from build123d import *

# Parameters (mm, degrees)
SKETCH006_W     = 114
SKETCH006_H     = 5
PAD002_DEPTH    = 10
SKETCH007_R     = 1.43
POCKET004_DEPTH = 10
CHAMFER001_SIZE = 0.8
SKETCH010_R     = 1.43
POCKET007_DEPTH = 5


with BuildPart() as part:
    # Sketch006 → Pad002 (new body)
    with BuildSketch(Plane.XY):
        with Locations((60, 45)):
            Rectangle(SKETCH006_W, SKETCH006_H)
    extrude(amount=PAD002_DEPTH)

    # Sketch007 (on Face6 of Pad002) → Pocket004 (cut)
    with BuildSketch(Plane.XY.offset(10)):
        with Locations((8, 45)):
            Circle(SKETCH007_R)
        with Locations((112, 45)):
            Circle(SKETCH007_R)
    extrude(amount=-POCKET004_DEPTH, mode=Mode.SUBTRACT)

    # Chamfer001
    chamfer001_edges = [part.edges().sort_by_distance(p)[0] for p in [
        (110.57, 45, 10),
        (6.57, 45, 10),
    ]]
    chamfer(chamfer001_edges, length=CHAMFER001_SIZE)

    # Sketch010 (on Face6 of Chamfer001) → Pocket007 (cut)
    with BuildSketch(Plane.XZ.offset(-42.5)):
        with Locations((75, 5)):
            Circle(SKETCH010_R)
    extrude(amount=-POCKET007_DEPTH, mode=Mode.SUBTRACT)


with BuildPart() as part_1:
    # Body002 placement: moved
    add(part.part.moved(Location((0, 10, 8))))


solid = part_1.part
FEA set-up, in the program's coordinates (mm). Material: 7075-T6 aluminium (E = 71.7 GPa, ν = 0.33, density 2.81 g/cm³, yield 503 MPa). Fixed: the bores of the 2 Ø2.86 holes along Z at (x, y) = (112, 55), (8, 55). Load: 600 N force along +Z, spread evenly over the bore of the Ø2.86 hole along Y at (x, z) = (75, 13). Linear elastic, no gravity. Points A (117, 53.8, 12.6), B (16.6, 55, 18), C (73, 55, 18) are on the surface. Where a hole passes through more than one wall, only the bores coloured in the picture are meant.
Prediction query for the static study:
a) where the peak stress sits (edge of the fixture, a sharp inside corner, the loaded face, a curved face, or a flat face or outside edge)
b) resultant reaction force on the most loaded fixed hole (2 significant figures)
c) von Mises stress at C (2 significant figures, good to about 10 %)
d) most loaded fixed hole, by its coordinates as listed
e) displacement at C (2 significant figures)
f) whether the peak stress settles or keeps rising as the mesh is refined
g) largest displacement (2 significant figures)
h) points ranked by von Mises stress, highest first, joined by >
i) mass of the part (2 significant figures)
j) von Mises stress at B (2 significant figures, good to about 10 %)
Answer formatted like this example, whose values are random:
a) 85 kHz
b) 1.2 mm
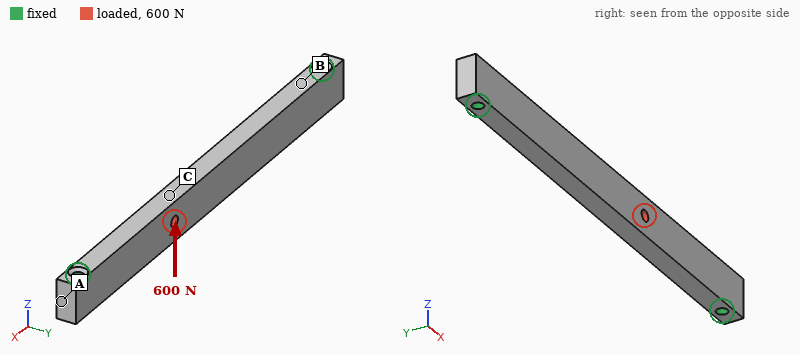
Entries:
a) edge of the fixture
b) 430 N
c) 80 MPa
d) (112, 55)
e) 0.10 mm
f) keeps rising
g) 0.11 mm
h) C > B > A
i) 16 g
j) 44 MPa
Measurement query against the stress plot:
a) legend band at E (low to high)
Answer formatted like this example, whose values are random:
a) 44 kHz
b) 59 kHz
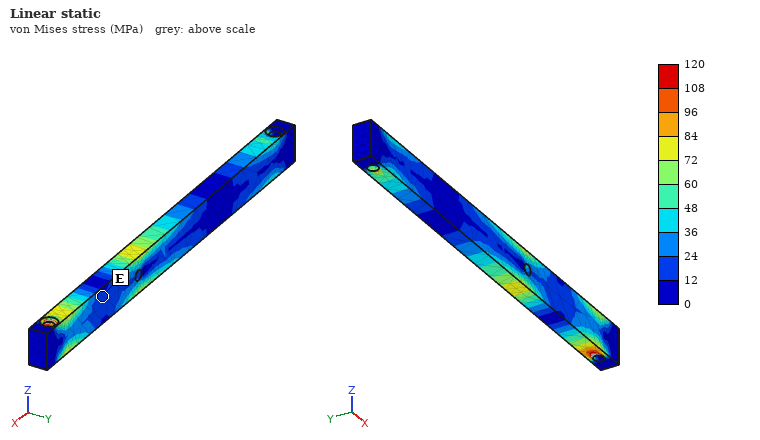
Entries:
a) 12 to 24 MPa
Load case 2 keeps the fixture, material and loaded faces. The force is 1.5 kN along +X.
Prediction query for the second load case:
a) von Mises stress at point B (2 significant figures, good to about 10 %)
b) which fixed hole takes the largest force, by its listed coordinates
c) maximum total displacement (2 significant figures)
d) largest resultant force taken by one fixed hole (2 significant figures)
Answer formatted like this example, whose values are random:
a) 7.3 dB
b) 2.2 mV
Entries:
a) 10 MPa
b) (112, 55)
c) 11 µm
d) 970 N
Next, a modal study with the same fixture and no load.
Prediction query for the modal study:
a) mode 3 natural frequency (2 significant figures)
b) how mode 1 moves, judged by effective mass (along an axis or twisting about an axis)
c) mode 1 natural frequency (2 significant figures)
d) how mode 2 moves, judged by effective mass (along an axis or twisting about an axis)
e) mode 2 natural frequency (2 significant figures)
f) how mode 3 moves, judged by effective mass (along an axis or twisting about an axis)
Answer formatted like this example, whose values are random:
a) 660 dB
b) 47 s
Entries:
a) 6400 Hz
b) along Y
c) 2400 Hz
d) along Z
e) 4600 Hz
f) twisting about Z
